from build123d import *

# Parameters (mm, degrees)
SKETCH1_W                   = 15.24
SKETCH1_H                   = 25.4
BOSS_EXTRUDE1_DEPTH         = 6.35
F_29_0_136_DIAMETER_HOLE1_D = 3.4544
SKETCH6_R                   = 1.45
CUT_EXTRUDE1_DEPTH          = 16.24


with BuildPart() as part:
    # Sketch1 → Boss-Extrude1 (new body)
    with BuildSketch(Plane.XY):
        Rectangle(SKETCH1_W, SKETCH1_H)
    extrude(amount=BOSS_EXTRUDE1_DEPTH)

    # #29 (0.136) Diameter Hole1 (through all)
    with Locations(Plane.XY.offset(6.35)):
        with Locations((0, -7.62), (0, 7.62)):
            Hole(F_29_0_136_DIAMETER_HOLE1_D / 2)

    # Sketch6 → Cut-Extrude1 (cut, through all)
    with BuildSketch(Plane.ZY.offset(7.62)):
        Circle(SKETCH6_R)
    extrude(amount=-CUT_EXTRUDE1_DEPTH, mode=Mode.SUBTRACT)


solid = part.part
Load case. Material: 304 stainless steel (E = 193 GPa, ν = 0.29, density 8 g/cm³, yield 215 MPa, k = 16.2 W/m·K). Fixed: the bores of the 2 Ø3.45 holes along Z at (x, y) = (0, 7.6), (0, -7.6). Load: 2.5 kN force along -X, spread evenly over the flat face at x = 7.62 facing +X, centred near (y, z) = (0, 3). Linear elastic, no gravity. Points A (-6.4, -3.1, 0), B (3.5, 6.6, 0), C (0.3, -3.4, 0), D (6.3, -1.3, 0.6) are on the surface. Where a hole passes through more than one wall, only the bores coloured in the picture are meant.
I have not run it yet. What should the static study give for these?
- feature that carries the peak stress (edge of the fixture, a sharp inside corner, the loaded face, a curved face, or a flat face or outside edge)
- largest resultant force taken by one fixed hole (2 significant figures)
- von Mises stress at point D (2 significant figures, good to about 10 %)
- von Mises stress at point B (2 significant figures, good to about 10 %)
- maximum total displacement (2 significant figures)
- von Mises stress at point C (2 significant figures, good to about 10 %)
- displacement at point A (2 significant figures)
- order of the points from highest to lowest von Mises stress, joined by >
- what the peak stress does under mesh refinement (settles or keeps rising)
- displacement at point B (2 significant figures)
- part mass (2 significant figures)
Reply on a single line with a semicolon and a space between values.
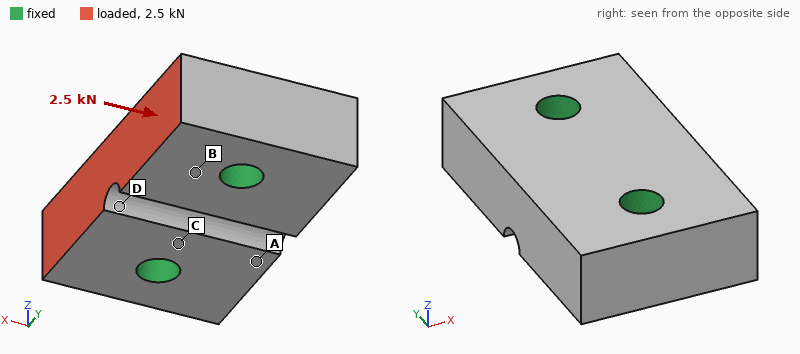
edge of the fixture; 1.3 kN; 14 MPa; 22 MPa; 0.92 µm; 8.0 MPa; 0.24 µm; B > D > C > A; keeps rising; 0.28 µm; 18 g
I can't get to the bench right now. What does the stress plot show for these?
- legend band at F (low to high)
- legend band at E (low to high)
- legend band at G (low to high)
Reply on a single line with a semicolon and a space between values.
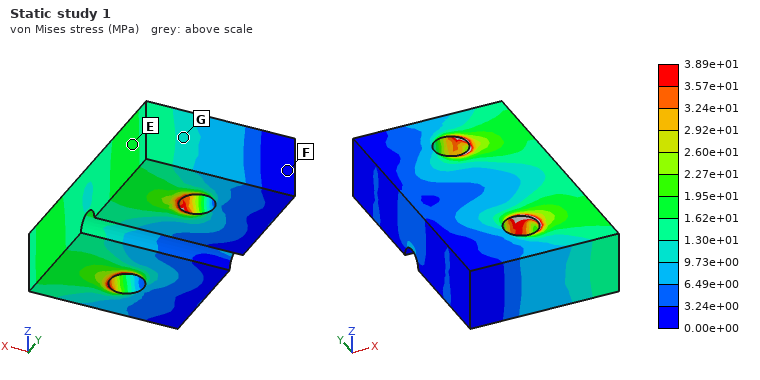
0.00e+00 to 3.24e+00 MPa; 1.62e+01 to 1.95e+01 MPa; 9.73e+00 to 1.30e+01 MPa
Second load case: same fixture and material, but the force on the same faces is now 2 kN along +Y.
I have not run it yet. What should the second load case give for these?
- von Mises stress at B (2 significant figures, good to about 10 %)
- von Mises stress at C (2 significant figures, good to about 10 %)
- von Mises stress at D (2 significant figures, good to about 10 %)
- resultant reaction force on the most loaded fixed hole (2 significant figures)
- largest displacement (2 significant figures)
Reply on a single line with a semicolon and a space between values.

28 MPa; 13 MPa; 26 MPa; 1.2 kN; 2.8 µm
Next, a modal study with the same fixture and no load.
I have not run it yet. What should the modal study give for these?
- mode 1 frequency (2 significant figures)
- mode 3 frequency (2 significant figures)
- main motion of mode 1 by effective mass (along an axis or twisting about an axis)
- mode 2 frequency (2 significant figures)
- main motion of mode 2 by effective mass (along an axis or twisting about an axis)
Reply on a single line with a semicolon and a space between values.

55 kHz; 71 kHz; twisting about Y; 62 kHz; along Z
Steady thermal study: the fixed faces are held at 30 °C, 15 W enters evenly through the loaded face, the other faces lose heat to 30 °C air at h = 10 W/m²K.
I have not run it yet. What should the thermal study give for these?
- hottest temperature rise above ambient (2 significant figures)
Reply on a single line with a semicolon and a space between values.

47 K
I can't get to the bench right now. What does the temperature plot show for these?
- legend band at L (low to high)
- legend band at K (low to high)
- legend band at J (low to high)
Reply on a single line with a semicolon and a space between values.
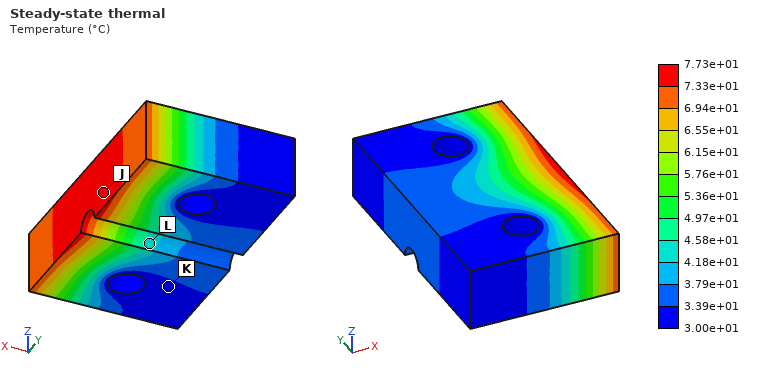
4.18e+01 to 4.58e+01 °C; 3.00e+01 to 3.39e+01 °C; 7.33e+01 to 7.73e+01 °C
